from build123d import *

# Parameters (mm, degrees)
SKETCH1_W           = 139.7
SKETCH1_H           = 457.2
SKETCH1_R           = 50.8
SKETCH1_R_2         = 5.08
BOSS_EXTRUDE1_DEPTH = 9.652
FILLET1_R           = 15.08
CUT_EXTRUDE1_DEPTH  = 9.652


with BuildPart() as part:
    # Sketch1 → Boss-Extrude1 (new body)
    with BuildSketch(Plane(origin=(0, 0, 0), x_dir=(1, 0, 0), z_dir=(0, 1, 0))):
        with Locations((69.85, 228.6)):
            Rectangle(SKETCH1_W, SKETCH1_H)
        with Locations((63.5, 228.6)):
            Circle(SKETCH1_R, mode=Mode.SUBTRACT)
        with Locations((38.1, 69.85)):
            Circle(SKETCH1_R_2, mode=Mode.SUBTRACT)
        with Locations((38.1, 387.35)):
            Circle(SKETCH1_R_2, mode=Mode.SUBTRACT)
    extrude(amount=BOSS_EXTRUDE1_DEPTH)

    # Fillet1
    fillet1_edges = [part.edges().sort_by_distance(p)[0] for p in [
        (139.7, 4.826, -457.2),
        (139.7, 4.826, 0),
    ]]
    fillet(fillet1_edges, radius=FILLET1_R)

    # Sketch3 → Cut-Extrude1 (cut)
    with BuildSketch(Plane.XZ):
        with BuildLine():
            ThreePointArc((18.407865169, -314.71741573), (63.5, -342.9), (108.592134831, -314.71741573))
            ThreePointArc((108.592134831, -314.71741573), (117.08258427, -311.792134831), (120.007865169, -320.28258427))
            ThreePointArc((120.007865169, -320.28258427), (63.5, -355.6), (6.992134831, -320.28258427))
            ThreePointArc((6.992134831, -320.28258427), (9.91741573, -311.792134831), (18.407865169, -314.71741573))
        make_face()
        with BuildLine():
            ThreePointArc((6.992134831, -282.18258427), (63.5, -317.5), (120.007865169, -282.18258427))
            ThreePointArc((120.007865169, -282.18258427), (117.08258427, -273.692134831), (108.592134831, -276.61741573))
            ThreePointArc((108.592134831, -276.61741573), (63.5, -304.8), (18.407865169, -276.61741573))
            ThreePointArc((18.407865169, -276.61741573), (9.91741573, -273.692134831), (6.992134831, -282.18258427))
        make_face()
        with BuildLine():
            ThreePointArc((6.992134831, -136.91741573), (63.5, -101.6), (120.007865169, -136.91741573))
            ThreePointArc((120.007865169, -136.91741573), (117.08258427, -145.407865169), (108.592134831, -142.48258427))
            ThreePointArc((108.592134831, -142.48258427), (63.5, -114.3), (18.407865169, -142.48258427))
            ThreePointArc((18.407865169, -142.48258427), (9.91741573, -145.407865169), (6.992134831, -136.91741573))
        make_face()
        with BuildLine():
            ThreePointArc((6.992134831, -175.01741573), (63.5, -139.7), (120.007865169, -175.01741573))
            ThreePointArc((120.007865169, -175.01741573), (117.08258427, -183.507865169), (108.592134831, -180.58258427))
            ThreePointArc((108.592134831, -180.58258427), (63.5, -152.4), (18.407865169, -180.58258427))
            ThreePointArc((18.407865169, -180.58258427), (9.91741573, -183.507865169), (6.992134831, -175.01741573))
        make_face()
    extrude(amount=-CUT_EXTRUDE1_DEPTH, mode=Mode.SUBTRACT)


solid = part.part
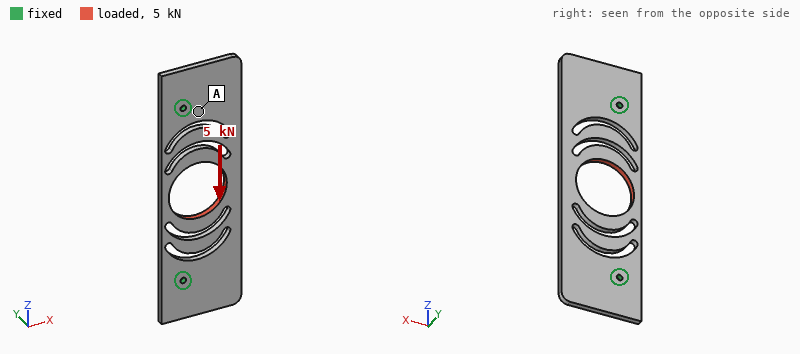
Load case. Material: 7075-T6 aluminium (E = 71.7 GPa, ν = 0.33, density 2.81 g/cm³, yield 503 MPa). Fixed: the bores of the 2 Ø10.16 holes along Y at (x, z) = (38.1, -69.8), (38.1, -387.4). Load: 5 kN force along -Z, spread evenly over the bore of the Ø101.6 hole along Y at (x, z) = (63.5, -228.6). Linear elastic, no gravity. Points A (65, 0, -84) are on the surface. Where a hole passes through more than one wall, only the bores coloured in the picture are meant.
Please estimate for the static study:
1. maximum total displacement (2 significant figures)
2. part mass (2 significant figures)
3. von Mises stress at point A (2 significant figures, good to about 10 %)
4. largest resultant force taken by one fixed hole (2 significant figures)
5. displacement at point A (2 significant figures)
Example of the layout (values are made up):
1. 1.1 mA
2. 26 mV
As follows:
1. 58 µm
2. 1.3 kg
3. 3.9 MPa
4. 2.5 kN
5. 12 µm
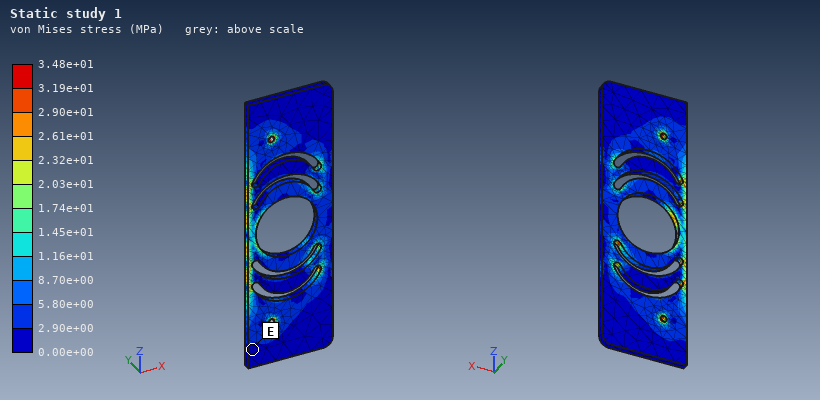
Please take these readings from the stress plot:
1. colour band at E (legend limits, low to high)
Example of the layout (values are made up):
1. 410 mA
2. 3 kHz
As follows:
1. 0.00e+00 to 2.90e+00 MPa
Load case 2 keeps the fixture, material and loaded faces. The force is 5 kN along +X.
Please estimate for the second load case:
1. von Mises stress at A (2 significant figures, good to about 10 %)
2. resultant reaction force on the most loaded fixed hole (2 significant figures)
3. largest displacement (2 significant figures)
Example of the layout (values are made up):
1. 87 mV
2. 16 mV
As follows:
1. 9.6 MPa
2. 2.9 kN
3. 0.25 mm
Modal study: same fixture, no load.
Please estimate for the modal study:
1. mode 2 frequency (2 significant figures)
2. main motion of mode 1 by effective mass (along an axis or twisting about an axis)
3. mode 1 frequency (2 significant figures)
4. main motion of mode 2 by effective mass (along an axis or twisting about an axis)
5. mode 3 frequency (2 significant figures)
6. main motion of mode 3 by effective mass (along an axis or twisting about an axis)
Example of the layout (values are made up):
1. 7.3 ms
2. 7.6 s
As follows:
1. 540 Hz
2. along Y
3. 340 Hz
4. twisting about Z
5. 590 Hz
6. twisting about X
